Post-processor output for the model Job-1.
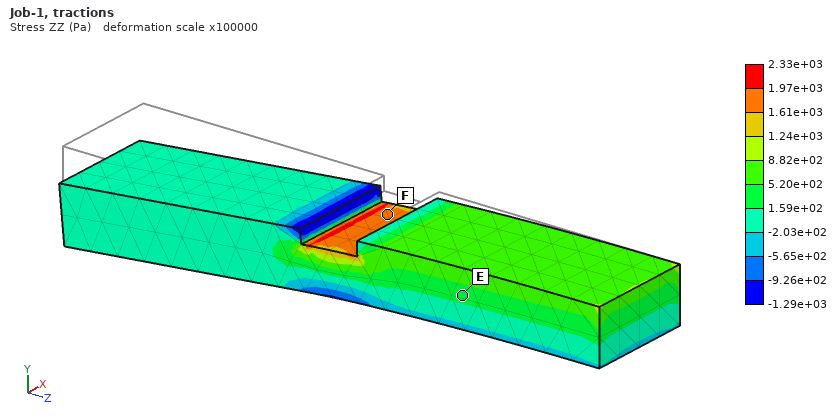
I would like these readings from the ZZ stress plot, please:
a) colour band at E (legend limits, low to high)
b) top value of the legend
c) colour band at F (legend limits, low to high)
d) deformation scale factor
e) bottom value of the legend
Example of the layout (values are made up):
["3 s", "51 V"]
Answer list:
["1.59e+02 to 5.20e+02 Pa", "2.33e+03 Pa", "1.61e+03 to 1.97e+03 Pa", "100000", "-1.29e+03 Pa"]
